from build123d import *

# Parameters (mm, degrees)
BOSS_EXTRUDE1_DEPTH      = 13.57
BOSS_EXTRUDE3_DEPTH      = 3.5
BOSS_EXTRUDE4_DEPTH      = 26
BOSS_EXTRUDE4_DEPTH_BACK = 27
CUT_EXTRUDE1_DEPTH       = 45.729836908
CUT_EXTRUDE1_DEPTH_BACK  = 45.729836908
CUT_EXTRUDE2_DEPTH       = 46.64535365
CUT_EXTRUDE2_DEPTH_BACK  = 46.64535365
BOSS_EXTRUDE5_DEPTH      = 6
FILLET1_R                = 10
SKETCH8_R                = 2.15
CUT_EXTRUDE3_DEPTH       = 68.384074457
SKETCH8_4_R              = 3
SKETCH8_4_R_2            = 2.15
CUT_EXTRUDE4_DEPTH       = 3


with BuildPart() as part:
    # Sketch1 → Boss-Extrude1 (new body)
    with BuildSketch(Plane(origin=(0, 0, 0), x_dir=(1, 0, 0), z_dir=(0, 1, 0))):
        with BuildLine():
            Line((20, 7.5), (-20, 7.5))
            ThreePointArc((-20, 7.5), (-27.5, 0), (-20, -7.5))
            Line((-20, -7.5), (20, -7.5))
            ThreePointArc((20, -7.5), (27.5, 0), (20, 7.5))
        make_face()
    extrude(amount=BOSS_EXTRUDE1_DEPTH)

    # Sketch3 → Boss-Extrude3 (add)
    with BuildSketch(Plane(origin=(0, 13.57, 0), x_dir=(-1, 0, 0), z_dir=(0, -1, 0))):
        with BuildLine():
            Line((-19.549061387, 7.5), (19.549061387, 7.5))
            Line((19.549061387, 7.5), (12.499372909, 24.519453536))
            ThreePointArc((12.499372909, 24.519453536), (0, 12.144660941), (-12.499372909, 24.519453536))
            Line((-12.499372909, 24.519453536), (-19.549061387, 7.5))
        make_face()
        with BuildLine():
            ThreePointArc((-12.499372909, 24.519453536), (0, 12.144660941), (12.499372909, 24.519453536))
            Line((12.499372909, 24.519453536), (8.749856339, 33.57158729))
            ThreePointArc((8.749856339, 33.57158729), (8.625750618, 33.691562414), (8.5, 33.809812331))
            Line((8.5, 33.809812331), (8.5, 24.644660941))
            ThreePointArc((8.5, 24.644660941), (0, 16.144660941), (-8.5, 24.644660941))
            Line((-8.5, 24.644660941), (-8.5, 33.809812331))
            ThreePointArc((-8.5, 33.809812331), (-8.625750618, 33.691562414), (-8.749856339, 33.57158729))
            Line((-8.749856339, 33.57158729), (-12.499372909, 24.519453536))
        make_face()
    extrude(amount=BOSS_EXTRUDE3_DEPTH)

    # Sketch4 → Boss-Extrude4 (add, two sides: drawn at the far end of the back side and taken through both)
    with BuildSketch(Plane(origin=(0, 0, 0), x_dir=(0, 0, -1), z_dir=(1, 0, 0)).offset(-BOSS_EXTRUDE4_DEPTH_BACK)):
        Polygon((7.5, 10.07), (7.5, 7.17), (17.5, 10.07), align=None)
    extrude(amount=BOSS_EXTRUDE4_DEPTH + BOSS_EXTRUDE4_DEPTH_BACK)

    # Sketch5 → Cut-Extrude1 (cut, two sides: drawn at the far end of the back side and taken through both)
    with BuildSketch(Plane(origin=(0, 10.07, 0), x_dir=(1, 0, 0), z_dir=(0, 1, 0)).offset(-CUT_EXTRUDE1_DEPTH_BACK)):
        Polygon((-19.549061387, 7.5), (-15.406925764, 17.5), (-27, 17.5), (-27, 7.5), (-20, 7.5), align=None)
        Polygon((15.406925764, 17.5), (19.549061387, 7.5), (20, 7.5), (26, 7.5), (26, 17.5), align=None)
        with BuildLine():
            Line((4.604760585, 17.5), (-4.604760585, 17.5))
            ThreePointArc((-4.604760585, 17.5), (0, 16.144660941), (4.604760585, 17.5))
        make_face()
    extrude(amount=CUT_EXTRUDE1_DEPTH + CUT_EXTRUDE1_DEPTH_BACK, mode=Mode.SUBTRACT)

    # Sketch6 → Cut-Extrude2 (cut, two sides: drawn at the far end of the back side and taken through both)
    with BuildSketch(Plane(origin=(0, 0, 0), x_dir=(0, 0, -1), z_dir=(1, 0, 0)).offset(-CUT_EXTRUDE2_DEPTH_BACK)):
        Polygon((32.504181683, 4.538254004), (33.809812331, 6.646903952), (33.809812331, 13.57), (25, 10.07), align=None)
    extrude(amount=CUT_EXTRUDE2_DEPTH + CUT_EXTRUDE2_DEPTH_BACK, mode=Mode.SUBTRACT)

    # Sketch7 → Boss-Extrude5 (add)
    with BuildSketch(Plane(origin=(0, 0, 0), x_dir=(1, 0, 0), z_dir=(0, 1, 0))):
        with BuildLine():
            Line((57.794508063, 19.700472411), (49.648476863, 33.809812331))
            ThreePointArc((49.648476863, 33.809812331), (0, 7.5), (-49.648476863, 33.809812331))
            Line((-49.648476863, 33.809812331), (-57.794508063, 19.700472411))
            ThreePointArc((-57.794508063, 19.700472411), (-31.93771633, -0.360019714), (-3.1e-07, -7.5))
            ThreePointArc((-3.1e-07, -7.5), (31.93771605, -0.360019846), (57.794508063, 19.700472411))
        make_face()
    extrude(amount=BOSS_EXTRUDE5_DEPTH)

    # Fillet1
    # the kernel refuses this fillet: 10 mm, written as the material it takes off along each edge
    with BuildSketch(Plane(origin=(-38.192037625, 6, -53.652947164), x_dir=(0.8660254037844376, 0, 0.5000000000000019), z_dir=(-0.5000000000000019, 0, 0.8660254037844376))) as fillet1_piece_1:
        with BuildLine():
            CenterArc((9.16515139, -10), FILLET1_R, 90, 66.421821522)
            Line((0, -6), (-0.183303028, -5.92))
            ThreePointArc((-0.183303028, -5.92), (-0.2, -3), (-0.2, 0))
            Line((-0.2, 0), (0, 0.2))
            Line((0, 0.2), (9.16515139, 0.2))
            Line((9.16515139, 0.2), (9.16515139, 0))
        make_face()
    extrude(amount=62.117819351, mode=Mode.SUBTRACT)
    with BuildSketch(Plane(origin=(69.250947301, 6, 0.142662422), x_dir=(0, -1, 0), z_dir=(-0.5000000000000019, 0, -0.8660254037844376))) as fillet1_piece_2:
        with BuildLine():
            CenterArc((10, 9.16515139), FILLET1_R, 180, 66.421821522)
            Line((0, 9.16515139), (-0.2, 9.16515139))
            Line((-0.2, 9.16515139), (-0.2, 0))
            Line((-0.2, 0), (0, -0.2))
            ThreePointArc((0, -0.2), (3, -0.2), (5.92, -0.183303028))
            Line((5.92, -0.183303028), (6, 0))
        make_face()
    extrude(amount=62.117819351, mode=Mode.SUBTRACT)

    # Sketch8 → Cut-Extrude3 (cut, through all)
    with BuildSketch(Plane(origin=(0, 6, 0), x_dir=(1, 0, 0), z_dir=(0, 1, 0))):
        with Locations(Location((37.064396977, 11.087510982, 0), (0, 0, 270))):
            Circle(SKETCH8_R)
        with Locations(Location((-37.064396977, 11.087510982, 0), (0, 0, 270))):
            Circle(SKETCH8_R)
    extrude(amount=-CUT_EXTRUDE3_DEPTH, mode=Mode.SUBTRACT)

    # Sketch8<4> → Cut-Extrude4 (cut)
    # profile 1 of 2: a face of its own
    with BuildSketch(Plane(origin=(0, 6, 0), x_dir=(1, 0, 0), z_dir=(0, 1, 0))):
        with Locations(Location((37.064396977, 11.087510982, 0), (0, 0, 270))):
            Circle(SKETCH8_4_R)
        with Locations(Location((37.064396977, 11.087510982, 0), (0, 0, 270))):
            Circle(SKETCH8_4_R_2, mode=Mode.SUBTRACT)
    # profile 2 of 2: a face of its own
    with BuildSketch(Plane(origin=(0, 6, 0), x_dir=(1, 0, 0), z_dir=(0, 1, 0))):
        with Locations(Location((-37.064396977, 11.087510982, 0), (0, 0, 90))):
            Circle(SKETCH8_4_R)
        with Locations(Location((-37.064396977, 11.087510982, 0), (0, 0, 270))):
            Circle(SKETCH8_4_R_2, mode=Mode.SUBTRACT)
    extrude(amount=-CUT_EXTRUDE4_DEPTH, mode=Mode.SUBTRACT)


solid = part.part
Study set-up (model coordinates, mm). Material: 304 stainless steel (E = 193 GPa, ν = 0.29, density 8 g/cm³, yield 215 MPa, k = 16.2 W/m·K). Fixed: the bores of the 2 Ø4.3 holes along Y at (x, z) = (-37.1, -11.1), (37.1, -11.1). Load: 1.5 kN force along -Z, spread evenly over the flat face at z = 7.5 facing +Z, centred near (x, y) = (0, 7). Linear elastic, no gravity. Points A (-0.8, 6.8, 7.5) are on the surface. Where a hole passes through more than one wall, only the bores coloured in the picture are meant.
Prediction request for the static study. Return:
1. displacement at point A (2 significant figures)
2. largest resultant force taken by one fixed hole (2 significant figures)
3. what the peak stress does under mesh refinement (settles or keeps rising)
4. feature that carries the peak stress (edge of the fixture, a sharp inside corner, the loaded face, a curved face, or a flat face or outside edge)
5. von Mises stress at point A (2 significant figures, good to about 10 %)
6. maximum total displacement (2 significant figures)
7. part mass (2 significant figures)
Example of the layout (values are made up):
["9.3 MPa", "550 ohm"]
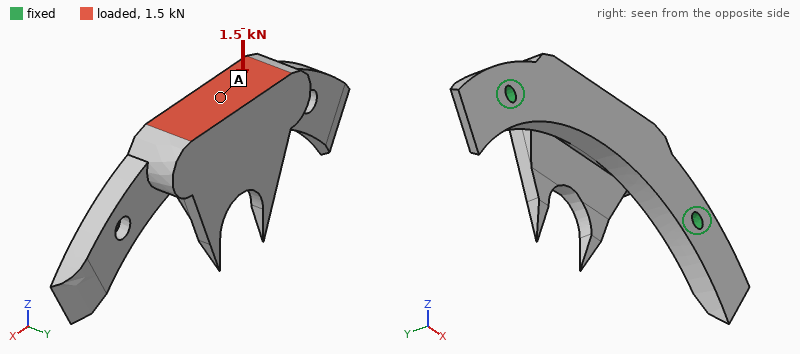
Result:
["24 µm", "1.0 kN", "keeps rising", "edge of the fixture", "14 MPa", "33 µm", "150 g"]
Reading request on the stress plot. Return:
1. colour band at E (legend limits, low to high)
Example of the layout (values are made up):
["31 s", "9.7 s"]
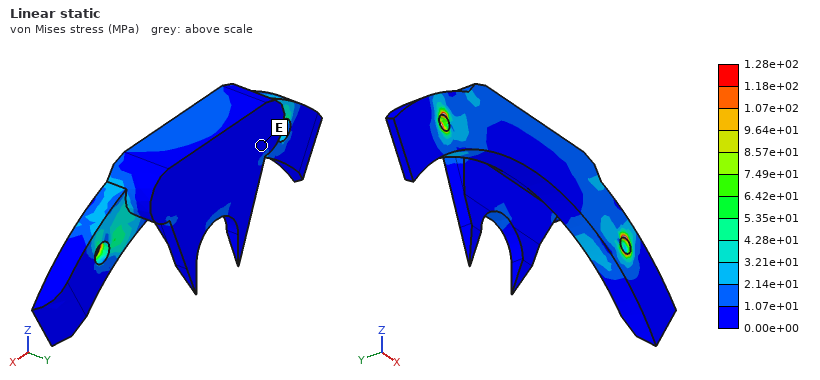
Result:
["0.00e+00 to 1.07e+01 MPa"]
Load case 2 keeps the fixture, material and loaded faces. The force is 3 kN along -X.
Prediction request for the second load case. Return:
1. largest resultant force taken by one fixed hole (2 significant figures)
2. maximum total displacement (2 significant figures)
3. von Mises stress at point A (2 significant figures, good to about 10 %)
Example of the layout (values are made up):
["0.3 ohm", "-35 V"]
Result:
["1.7 kN", "3.8 µm", "12 MPa"]
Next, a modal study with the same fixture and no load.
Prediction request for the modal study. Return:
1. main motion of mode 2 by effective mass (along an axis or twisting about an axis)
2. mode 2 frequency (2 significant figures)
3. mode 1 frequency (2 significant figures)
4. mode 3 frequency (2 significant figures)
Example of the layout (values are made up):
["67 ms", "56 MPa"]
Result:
["along Y", "5900 Hz", "3000 Hz", "7800 Hz"]
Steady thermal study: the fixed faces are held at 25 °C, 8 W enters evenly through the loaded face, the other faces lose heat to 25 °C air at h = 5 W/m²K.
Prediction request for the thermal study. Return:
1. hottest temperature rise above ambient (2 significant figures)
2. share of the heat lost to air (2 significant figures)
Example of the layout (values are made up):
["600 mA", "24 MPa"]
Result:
["63 K", "14 %"]
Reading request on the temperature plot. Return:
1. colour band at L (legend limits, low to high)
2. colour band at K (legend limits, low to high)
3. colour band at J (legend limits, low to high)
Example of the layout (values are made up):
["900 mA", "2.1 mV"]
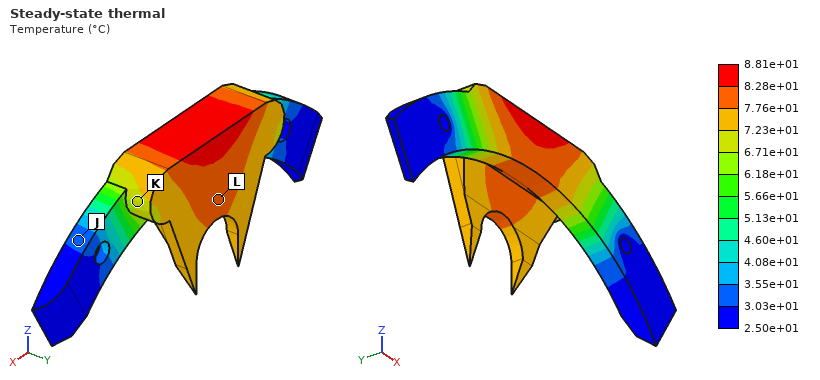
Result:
["7.76e+01 to 8.28e+01 °C", "6.71e+01 to 7.23e+01 °C", "3.03e+01 to 3.55e+01 °C"]
